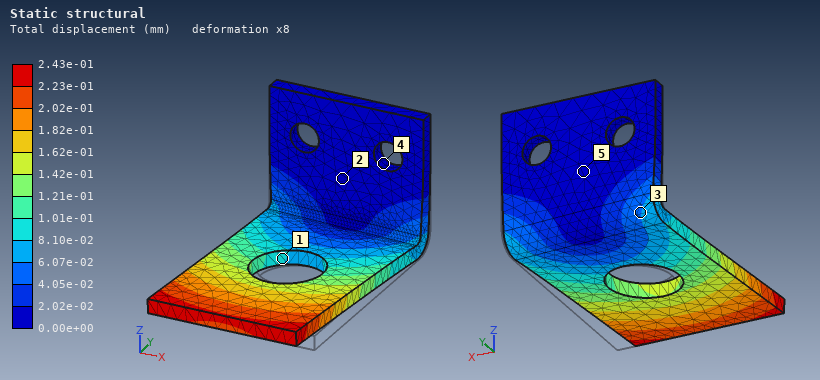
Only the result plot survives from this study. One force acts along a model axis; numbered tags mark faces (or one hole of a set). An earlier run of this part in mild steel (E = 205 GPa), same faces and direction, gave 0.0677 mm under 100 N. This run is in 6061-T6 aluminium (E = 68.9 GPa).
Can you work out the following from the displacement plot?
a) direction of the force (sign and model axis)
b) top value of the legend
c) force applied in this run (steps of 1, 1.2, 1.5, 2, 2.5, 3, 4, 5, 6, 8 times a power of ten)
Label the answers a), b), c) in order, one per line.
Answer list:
a) -X
b) 2.43e-01 mm
c) 120 N
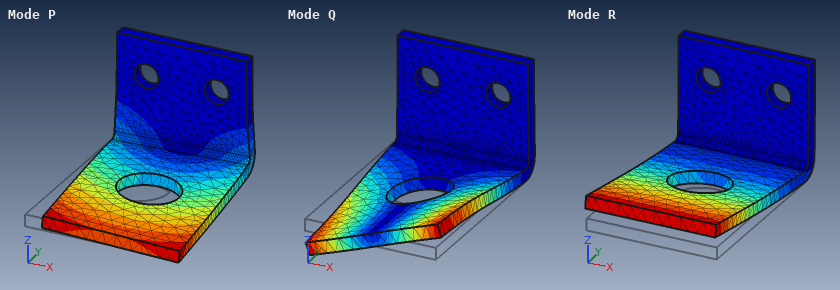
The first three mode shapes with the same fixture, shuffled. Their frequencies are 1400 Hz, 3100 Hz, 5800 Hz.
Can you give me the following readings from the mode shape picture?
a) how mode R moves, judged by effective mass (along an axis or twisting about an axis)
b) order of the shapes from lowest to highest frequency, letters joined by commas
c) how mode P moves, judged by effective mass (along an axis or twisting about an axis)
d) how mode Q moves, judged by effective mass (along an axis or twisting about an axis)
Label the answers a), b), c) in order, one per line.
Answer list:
a) along Z
b) R, P, Q
c) along X
d) twisting about Y
